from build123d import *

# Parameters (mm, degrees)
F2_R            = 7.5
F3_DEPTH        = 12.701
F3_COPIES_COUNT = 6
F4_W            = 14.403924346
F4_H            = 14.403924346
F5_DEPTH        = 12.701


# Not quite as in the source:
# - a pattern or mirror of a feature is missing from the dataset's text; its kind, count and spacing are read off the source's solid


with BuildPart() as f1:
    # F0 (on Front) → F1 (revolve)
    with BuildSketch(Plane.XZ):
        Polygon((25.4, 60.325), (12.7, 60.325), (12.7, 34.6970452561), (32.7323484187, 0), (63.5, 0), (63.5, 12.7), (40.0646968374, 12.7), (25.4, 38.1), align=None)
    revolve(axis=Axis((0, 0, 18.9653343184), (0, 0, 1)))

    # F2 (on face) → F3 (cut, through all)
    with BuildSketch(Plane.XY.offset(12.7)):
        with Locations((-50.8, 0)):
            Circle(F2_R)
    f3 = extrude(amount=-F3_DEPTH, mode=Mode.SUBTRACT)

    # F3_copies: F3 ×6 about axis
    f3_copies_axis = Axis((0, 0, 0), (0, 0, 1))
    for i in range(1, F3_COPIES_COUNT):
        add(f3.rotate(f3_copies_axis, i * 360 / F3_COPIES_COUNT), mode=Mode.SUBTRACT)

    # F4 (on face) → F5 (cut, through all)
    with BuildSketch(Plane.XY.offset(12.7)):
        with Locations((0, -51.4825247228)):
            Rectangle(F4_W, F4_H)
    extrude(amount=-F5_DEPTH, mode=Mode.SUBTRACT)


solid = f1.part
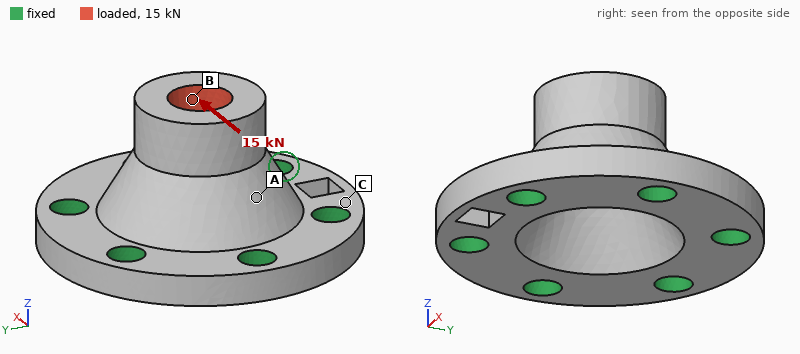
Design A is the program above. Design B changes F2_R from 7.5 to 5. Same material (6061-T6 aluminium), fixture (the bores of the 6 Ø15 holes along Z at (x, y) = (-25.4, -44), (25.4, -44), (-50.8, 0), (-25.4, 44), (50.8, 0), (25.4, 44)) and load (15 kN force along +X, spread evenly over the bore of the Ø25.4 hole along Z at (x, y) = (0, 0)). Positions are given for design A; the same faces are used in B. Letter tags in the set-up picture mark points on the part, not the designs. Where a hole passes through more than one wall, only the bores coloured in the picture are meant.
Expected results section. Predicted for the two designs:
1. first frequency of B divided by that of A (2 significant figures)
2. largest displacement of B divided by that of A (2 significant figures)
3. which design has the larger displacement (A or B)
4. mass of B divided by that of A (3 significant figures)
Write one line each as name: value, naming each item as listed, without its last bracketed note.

first frequency of B divided by that of A: 0.90
largest displacement of B divided by that of A: 1.1
which design has the larger displacement: B
mass of B divided by that of A: 1.04
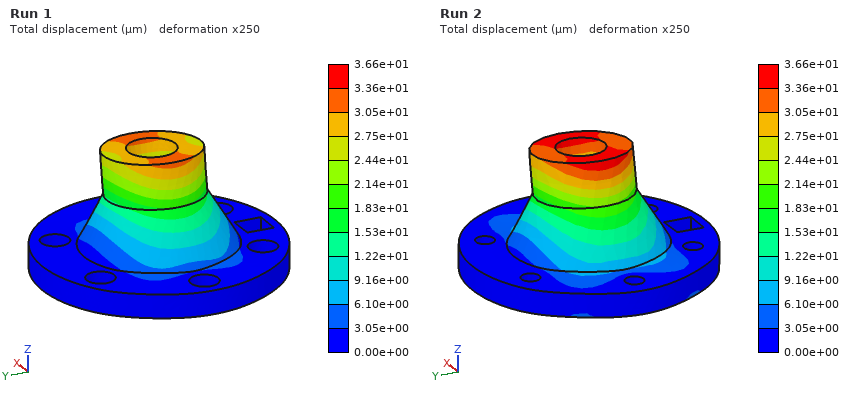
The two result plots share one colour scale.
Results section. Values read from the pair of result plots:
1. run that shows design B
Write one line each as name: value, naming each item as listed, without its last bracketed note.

run that shows design B: Run 2
